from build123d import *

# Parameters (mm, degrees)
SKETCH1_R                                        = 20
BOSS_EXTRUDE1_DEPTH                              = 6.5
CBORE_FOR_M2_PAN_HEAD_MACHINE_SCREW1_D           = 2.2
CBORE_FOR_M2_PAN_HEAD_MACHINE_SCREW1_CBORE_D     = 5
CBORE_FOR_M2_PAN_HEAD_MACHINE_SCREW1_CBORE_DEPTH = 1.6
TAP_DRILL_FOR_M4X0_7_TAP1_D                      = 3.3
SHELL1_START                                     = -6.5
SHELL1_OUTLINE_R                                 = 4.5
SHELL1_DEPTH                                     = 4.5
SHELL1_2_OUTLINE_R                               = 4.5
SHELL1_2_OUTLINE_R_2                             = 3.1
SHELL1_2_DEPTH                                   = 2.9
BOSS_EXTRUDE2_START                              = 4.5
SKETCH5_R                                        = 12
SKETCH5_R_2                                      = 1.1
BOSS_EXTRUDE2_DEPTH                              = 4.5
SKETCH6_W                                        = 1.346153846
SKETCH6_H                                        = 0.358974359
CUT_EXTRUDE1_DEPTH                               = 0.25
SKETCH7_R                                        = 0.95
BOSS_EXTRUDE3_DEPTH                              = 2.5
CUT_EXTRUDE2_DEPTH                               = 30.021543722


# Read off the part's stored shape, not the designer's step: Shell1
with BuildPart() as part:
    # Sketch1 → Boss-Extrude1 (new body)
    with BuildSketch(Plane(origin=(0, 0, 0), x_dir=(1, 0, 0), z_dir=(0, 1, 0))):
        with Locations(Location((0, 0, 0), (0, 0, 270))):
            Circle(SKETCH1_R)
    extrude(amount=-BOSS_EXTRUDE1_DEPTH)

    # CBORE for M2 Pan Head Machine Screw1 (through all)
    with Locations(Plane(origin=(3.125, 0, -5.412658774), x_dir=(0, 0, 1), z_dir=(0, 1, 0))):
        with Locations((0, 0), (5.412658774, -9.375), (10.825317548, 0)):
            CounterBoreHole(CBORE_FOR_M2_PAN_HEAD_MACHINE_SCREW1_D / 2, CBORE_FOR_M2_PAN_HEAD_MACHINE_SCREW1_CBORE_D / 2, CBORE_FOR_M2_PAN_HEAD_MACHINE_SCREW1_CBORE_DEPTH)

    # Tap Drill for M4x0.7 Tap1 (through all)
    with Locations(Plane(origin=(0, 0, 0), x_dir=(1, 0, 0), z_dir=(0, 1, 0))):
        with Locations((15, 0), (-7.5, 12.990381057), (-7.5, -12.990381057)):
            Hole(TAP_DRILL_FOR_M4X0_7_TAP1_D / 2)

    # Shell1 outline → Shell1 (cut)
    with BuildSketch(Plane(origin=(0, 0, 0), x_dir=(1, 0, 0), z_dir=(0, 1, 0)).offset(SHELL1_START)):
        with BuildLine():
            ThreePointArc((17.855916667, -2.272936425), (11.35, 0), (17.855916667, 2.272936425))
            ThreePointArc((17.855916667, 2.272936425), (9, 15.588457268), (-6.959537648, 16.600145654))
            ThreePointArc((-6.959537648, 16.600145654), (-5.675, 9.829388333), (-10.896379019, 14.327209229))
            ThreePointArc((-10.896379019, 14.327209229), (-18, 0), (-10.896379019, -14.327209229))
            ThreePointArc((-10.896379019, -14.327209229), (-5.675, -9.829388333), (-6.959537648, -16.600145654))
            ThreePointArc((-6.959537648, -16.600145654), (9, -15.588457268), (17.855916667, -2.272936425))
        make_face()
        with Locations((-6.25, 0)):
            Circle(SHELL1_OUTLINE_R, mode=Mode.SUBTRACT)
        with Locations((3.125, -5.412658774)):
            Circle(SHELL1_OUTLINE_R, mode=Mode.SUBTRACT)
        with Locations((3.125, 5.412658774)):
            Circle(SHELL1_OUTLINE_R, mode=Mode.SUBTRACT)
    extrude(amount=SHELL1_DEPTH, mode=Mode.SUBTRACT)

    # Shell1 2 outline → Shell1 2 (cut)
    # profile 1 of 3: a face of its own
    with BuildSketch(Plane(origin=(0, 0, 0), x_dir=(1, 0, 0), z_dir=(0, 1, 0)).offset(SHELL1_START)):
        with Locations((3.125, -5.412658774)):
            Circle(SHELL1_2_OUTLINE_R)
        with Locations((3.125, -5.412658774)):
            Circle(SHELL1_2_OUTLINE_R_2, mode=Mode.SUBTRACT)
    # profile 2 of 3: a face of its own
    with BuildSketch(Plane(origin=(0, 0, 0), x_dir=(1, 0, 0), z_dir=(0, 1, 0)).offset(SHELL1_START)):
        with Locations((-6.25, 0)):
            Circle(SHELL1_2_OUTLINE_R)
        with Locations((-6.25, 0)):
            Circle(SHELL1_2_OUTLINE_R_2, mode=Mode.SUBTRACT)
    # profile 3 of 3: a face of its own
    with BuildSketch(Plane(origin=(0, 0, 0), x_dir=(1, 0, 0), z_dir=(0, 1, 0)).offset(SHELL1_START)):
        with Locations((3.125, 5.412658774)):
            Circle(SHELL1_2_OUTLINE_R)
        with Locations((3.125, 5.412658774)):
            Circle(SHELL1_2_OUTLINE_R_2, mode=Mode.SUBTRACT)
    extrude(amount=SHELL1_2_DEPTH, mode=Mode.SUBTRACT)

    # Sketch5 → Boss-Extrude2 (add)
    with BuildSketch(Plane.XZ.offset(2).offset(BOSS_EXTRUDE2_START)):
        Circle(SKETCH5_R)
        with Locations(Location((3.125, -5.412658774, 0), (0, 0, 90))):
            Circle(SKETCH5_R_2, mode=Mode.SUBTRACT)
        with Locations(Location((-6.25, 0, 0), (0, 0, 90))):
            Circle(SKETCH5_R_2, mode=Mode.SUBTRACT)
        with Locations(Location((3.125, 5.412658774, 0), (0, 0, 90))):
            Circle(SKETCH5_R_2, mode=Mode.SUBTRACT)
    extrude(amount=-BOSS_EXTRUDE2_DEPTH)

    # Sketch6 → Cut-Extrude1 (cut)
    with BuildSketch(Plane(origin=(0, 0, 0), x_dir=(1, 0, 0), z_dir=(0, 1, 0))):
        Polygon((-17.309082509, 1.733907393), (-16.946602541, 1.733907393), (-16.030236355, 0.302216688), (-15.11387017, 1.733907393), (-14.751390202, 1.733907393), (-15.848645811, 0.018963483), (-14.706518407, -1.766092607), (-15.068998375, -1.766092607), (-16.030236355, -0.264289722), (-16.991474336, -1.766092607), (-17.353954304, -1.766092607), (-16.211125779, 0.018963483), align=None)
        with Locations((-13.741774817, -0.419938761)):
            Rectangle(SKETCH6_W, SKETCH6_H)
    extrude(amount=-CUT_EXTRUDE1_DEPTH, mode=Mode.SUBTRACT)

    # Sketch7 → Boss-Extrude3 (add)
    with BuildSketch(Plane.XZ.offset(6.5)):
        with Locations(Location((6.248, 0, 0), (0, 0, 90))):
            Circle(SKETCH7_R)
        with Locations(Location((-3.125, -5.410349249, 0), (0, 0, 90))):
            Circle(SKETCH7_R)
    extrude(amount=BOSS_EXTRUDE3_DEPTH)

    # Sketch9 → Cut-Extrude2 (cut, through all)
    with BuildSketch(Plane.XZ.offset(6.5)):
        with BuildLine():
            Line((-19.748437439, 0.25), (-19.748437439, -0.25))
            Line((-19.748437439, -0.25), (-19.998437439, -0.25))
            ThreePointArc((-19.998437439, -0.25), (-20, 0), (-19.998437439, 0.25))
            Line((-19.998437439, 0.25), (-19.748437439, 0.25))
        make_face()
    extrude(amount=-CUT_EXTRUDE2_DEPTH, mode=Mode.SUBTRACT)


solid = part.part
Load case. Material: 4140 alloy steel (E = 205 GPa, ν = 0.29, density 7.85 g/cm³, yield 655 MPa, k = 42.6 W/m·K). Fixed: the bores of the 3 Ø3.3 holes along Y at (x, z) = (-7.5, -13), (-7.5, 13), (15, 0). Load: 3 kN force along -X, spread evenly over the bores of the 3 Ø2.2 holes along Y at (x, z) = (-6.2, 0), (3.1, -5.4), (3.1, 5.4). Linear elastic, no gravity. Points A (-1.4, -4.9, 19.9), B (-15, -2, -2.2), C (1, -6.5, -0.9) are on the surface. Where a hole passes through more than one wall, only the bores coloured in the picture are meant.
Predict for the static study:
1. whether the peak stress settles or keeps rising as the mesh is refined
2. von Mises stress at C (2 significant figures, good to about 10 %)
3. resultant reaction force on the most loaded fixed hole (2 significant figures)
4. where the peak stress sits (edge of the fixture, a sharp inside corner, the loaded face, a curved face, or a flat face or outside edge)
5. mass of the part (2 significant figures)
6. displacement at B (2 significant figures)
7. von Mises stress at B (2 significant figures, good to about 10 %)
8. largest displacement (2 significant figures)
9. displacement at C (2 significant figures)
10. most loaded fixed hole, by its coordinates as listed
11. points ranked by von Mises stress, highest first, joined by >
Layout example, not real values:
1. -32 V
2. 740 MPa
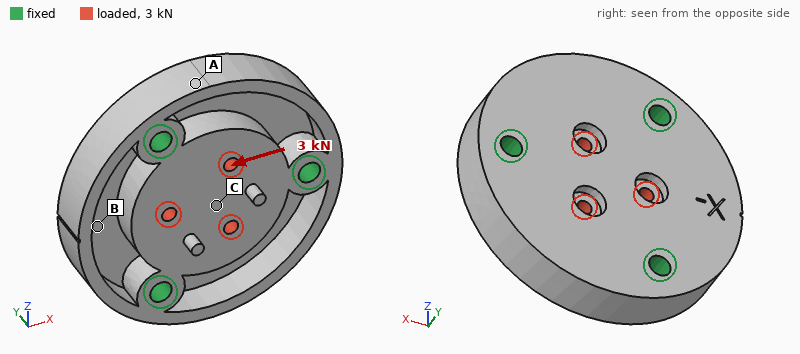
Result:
1. keeps rising
2. 22 MPa
3. 1.2 kN
4. edge of the fixture
5. 46 g
6. 1.3 µm
7. 13 MPa
8. 2.3 µm
9. 1.4 µm
10. (15, 0)
11. C > B > A
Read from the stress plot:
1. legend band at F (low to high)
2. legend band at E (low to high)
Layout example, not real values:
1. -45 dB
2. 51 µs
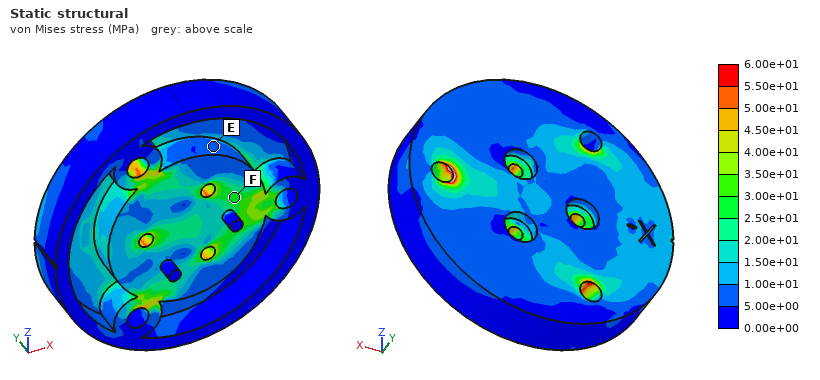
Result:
1. 2.50e+01 to 3.00e+01 MPa
2. 5.00e+00 to 1.00e+01 MPa
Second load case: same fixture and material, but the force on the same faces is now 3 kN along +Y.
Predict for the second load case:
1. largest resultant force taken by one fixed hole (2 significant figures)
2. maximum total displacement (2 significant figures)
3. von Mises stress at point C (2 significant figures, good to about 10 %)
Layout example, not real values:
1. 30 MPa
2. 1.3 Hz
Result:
1. 1.0 kN
2. 5.6 µm
3. 32 MPa
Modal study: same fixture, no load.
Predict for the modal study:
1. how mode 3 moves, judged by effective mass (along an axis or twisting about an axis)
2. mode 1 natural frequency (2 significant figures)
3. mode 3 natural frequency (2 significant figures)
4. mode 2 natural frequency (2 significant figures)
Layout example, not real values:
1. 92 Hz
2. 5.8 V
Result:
1. along Y
2. 19 kHz
3. 21 kHz
4. 19 kHz
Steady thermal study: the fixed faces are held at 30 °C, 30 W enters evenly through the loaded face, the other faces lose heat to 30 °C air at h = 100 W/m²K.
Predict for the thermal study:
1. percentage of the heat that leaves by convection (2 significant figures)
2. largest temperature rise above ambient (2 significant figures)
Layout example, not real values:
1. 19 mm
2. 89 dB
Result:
1. 17 %
2. 36 K
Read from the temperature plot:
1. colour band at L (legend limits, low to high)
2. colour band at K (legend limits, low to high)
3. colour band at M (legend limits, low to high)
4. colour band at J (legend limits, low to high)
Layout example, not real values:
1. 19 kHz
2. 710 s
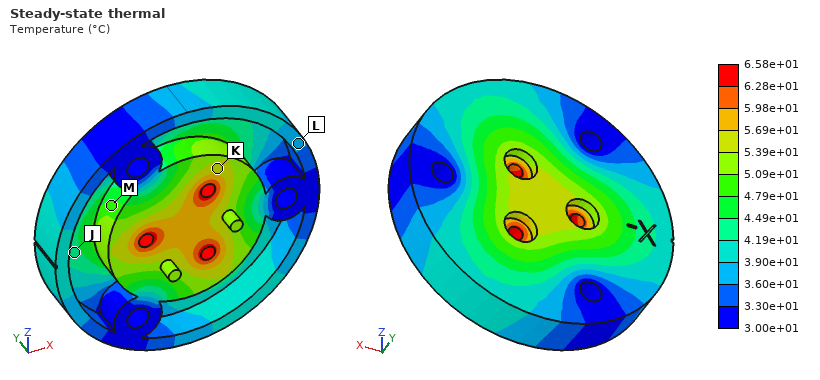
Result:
1. 3.60e+01 to 3.90e+01 °C
2. 5.39e+01 to 5.69e+01 °C
3. 4.79e+01 to 5.09e+01 °C
4. 4.19e+01 to 4.49e+01 °C
